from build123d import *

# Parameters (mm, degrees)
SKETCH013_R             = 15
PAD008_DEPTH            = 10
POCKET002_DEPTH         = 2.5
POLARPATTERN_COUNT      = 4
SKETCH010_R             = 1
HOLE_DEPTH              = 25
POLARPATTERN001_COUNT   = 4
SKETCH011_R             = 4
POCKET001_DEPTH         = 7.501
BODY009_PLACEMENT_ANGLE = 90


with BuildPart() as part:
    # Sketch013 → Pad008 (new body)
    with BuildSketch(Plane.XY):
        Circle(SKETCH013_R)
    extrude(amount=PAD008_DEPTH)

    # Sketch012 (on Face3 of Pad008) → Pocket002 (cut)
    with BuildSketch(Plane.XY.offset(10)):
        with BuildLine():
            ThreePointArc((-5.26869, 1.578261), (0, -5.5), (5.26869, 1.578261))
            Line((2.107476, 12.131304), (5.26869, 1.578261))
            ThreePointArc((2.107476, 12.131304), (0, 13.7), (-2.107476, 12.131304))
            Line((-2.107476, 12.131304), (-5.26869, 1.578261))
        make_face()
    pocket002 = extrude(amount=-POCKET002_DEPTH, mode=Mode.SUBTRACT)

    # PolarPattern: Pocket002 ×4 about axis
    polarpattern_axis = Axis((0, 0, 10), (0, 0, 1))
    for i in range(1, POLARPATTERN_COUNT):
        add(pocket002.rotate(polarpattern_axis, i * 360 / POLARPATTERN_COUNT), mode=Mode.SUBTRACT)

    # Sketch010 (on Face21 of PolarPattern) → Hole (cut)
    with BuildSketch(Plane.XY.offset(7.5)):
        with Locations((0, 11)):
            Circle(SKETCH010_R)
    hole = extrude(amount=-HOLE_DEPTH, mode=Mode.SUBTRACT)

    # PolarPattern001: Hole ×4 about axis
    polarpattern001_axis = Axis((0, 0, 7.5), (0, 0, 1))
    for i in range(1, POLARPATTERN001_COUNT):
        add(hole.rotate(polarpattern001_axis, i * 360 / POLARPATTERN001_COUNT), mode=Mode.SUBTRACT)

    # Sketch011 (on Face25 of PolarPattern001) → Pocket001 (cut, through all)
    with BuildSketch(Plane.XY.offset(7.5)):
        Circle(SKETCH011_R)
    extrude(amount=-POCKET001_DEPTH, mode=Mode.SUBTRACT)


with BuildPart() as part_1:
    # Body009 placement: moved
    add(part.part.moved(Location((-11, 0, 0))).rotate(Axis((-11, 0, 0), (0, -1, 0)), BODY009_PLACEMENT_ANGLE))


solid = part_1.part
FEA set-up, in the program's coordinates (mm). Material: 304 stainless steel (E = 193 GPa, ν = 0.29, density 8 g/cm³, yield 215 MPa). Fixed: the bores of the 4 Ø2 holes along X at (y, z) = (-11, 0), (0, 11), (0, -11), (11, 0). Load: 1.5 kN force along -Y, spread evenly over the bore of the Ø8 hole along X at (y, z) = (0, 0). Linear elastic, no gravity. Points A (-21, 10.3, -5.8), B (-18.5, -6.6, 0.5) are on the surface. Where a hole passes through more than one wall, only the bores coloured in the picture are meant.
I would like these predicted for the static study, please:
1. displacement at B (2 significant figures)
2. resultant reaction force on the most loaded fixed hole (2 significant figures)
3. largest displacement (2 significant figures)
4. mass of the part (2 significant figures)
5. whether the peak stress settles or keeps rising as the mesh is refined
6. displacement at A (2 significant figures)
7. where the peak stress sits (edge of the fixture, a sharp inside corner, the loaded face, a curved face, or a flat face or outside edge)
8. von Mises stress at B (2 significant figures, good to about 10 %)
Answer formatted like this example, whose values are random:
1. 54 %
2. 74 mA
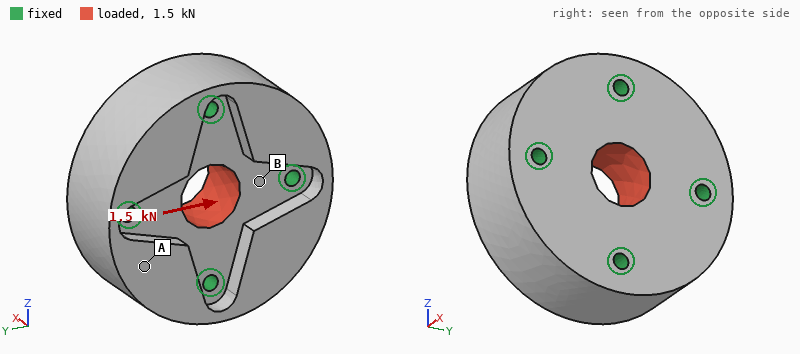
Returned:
1. 0.22 µm
2. 460 N
3. 0.42 µm
4. 47 g
5. keeps rising
6. 0.19 µm
7. edge of the fixture
8. 10 MPa
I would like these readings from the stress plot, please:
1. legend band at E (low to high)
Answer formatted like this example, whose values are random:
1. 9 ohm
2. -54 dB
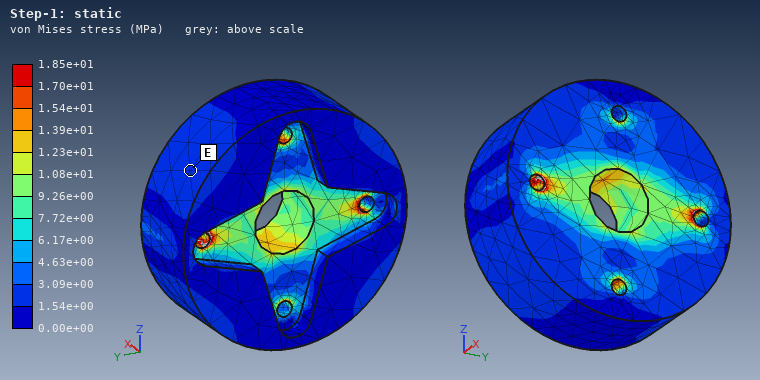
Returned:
1. 1.54e+00 to 3.09e+00 MPa
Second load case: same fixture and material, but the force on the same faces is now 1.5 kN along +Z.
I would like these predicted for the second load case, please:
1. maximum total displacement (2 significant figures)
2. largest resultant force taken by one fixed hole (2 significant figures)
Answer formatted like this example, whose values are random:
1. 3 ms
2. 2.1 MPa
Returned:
1. 0.41 µm
2. 460 N
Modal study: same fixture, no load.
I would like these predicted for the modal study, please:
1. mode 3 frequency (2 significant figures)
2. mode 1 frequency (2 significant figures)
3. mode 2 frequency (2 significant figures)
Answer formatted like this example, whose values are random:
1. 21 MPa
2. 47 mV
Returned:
1. 51 kHz
2. 48 kHz
3. 51 kHz
